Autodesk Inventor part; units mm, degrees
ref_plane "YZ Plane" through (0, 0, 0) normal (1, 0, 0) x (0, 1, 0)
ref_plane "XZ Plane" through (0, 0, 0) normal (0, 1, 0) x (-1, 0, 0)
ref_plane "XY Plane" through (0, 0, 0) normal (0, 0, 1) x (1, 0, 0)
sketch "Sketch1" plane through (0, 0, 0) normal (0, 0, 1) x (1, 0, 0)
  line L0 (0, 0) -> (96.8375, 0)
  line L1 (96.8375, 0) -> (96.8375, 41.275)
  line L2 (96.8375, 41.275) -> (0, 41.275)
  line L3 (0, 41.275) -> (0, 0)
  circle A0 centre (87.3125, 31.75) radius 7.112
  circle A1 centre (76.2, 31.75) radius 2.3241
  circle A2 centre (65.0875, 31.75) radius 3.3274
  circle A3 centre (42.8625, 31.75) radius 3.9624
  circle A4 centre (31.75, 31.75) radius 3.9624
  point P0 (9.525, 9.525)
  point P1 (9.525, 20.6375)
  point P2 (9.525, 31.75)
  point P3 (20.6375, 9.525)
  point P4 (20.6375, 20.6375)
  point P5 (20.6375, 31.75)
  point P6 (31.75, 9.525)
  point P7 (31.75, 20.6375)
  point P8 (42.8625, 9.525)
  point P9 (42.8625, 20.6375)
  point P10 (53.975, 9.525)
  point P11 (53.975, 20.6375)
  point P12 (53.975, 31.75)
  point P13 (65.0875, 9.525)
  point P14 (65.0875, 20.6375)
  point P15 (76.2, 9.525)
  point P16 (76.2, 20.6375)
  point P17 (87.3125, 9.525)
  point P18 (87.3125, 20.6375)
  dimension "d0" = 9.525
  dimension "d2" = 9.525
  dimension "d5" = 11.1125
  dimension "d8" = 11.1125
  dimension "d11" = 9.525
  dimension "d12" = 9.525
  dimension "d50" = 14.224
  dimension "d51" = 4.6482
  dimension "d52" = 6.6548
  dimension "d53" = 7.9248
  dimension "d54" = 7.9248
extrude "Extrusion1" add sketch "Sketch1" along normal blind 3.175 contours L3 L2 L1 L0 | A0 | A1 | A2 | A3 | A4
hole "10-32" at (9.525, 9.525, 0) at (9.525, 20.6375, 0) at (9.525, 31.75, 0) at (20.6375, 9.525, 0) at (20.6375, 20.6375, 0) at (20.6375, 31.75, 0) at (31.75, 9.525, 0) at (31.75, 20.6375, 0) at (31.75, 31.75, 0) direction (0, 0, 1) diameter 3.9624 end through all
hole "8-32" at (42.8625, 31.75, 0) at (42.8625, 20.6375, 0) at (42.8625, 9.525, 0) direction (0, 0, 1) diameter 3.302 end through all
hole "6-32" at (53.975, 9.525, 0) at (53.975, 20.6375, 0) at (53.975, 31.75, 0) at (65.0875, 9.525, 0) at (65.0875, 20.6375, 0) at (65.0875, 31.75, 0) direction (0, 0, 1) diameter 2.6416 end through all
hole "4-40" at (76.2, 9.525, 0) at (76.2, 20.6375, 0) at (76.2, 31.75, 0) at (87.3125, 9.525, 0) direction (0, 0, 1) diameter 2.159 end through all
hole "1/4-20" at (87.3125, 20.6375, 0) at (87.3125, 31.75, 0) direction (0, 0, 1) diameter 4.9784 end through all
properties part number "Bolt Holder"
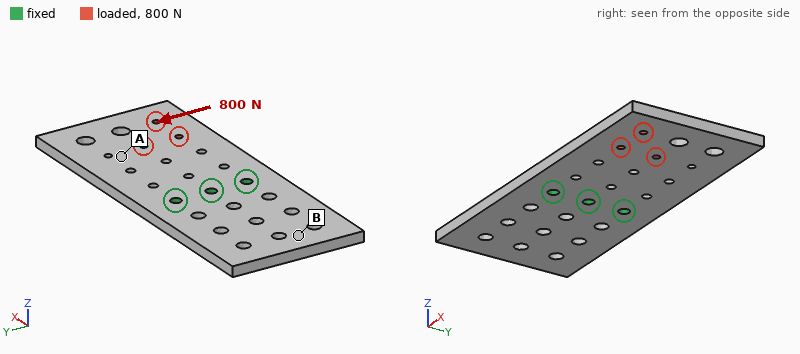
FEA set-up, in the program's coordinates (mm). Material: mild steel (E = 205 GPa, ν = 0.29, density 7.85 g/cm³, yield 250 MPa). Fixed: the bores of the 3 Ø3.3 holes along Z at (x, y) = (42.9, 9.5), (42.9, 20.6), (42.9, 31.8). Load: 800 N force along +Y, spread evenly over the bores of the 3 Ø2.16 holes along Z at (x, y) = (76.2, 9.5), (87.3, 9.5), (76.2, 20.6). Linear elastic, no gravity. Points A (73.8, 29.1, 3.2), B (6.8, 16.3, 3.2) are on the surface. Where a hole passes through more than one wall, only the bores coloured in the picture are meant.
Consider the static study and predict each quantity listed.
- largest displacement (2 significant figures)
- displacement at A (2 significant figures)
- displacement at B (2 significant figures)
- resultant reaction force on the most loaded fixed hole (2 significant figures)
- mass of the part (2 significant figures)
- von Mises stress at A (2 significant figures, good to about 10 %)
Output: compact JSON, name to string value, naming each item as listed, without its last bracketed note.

{"largest displacement": "14 µm", "displacement at A": "7.8 µm", "displacement at B": "2.4 µm", "resultant reaction force on the most loaded fixed hole": "1.2 kN", "mass of the part": "94 g", "von Mises stress at A": "10.0 MPa"}
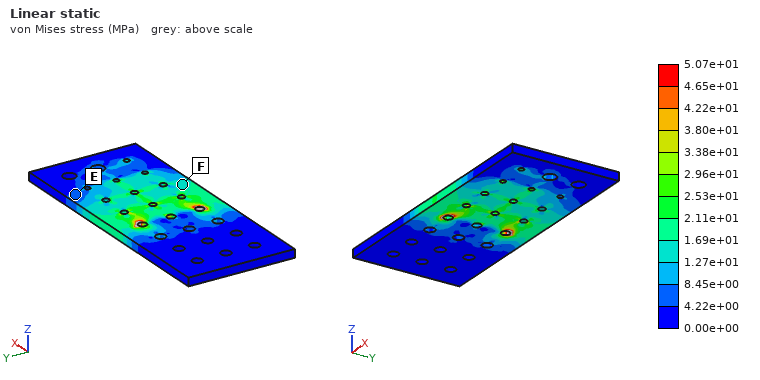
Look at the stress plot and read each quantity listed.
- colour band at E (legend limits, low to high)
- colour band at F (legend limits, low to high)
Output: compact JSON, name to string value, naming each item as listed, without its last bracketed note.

{"colour band at E": "4.22e+00 to 8.45e+00 MPa", "colour band at F": "1.27e+01 to 1.69e+01 MPa"}
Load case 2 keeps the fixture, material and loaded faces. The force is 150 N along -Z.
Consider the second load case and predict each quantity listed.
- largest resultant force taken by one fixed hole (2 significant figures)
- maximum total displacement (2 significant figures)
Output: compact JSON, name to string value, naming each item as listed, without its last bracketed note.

{"largest resultant force taken by one fixed hole": "77 N", "maximum total displacement": "0.21 mm"}
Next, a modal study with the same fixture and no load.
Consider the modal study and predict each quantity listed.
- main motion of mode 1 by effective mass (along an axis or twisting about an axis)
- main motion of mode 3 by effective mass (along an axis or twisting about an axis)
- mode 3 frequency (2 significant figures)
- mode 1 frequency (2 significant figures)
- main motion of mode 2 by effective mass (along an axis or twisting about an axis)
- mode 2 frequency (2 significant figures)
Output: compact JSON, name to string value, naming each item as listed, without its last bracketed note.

{"main motion of mode 1 by effective mass": "along Z", "main motion of mode 3 by effective mass": "twisting about X", "mode 3 frequency": "2600 Hz", "mode 1 frequency": "920 Hz", "main motion of mode 2 by effective mass": "along Z", "mode 2 frequency": "1400 Hz"}
